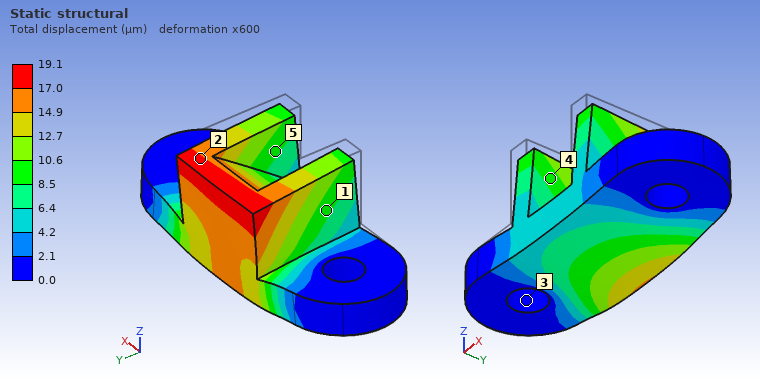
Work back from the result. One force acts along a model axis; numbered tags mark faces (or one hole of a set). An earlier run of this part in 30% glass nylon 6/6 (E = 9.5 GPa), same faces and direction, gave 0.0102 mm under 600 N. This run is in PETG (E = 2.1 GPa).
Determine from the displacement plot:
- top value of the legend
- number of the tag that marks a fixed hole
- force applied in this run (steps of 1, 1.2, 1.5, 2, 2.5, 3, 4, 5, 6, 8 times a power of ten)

19.1 µm
3
250 N
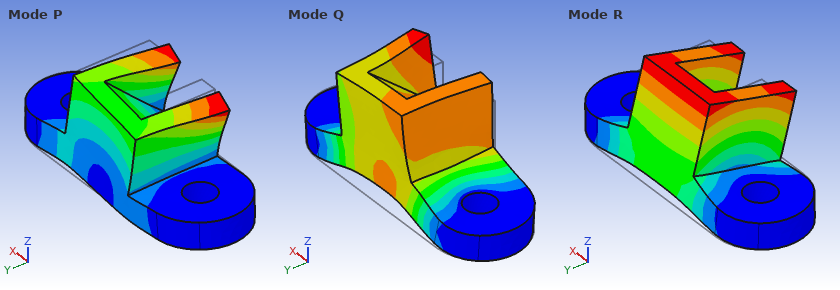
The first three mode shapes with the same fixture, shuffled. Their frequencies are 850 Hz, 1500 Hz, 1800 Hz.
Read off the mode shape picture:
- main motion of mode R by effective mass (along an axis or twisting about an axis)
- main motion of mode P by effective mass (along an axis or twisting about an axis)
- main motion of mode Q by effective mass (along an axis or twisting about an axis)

along Y
along X
along Z
